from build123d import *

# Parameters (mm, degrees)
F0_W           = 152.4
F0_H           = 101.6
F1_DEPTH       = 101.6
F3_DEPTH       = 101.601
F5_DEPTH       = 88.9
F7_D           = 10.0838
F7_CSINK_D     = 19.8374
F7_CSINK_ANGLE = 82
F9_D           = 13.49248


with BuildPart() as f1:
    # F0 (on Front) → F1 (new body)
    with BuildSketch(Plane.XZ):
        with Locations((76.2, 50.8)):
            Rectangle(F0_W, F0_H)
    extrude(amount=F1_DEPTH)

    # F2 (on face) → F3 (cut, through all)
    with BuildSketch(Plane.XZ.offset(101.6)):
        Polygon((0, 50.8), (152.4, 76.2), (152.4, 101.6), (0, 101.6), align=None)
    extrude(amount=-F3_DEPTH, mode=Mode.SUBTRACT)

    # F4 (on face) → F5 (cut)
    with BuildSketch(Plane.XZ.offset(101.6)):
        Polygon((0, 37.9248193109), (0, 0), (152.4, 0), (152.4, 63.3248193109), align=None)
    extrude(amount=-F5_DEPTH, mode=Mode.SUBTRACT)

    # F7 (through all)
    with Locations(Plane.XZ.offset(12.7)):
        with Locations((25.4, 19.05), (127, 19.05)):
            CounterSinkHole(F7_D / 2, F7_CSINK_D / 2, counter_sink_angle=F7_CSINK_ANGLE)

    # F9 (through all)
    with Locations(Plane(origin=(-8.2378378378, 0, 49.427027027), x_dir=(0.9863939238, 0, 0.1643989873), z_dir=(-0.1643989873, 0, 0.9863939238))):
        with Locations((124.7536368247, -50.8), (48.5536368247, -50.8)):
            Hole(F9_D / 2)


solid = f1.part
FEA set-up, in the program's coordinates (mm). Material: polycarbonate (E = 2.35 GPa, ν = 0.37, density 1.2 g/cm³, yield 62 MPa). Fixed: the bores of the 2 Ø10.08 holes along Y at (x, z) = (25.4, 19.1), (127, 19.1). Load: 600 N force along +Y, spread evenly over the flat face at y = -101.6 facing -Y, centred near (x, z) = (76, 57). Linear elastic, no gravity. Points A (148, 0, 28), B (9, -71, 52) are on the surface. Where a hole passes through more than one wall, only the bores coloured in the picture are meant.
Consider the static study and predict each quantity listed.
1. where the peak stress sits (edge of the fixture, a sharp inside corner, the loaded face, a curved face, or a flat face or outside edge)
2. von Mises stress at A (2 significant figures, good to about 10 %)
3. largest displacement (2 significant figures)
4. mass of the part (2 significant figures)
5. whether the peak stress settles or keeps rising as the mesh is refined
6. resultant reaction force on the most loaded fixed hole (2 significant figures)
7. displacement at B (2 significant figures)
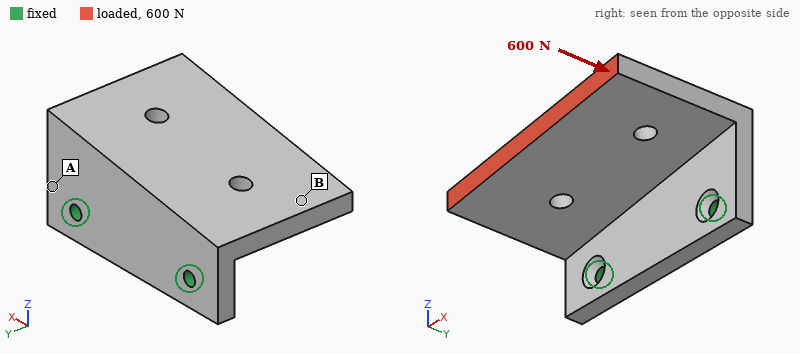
edge of the fixture
4.7 MPa
1.8 mm
350 g
keeps rising
300 N
0.99 mm
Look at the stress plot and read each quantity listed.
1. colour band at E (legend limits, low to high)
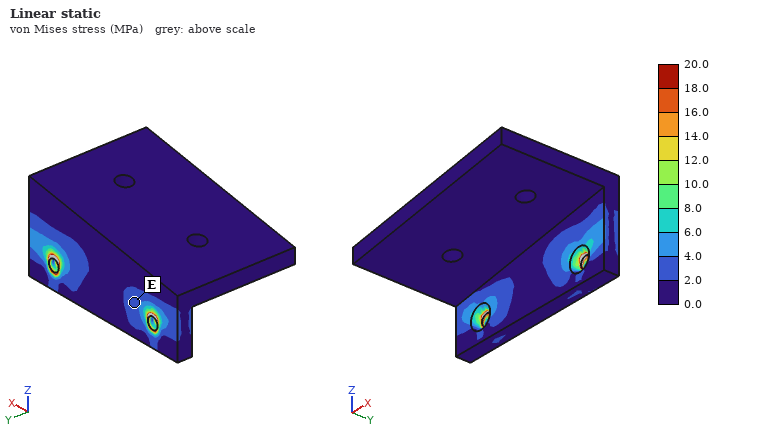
2.0 to 4.0 MPa
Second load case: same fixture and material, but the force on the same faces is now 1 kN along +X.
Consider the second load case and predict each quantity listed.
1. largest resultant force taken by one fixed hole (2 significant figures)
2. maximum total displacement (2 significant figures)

1.1 kN
2.3 mm
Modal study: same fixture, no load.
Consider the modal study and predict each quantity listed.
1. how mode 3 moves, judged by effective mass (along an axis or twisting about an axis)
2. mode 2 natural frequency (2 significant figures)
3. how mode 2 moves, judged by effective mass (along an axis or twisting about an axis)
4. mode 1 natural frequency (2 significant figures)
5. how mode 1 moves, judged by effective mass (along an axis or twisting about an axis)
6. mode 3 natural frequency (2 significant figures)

along Y
350 Hz
along X
160 Hz
along Z
510 Hz
